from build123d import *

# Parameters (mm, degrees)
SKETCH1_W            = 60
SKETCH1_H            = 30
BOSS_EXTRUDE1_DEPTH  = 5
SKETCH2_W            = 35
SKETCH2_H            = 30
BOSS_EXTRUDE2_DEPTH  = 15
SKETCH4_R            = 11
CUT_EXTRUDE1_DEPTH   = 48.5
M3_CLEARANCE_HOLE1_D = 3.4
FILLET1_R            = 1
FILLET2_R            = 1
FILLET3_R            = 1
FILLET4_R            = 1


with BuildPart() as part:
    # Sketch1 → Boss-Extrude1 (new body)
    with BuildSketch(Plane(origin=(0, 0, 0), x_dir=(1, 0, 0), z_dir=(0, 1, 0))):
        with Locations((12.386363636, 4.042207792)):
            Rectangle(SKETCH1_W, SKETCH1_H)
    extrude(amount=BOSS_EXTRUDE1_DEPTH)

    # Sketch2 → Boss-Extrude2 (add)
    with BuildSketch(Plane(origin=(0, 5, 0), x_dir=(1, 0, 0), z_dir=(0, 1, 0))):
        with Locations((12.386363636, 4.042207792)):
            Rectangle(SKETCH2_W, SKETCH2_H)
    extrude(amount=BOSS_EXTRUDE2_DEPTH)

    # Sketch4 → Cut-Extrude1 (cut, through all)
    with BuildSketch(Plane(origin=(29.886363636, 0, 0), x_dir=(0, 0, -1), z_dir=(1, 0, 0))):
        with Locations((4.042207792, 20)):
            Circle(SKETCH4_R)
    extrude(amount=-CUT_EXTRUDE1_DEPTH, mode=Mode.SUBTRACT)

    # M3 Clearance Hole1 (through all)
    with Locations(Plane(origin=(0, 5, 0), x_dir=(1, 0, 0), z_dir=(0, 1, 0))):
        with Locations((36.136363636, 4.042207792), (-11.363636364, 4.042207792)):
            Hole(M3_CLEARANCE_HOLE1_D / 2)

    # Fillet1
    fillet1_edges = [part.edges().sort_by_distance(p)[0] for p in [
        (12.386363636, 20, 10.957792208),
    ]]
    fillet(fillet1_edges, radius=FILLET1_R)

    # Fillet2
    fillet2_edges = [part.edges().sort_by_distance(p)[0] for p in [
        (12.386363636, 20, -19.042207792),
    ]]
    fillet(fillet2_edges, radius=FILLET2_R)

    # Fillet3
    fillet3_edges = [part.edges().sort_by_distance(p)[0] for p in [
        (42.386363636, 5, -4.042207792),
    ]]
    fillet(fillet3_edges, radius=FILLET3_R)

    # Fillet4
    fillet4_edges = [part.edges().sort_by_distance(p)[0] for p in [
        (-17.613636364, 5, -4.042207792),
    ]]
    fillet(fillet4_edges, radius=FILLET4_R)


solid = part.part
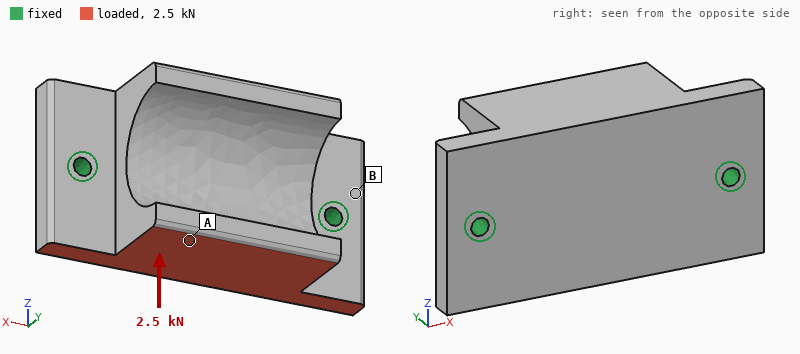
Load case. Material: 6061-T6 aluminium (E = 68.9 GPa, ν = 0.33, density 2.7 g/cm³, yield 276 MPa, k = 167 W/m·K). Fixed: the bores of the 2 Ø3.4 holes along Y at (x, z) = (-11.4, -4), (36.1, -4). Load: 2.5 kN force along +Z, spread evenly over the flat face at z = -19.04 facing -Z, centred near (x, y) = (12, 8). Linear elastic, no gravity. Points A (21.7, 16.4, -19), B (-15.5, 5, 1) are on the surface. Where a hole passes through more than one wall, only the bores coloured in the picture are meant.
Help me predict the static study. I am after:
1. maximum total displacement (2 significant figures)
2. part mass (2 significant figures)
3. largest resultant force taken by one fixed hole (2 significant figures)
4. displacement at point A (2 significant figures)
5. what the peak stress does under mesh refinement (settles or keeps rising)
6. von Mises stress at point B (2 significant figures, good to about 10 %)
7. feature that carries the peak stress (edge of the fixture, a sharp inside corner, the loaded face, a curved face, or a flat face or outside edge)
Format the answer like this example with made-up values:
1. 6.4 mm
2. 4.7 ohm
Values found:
1. 74 µm
2. 49 g
3. 1.3 kN
4. 65 µm
5. keeps rising
6. 30 MPa
7. edge of the fixture
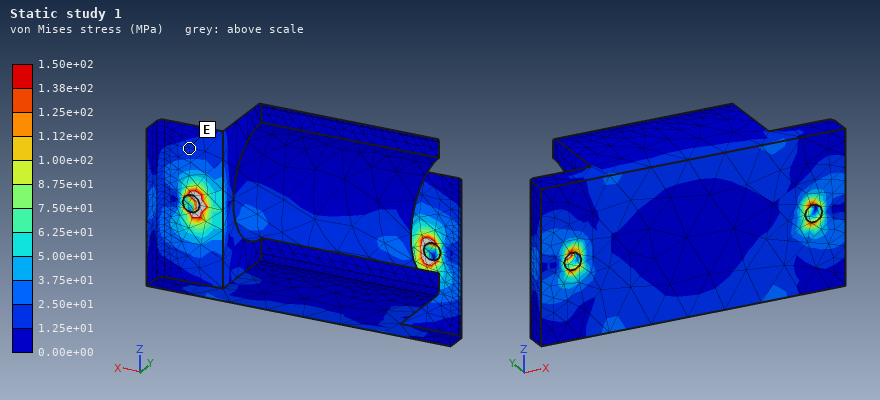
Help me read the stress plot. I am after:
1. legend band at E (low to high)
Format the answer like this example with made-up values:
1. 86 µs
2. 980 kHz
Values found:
1. 1.25e+01 to 2.50e+01 MPa
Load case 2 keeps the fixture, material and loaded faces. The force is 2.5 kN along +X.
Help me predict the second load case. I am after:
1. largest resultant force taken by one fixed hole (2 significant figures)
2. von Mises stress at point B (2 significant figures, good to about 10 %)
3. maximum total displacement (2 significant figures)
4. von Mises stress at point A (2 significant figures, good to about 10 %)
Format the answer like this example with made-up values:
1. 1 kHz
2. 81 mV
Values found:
1. 1.5 kN
2. 6.1 MPa
3. 11 µm
4. 8.3 MPa
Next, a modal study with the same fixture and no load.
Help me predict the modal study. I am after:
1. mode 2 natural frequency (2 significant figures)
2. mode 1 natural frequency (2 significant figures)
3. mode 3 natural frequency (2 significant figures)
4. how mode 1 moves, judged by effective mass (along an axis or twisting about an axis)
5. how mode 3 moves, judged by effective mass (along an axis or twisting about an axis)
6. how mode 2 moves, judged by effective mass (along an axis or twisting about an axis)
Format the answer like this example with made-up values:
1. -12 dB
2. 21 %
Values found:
1. 9600 Hz
2. 4900 Hz
3. 16 kHz
4. along Z
5. along X
6. along Y
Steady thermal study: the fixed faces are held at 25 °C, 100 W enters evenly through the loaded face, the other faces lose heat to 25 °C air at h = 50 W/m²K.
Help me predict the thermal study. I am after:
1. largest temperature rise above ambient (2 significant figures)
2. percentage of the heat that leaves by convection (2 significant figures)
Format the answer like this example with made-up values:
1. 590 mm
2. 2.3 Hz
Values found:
1. 45 K
2. 6.4 %
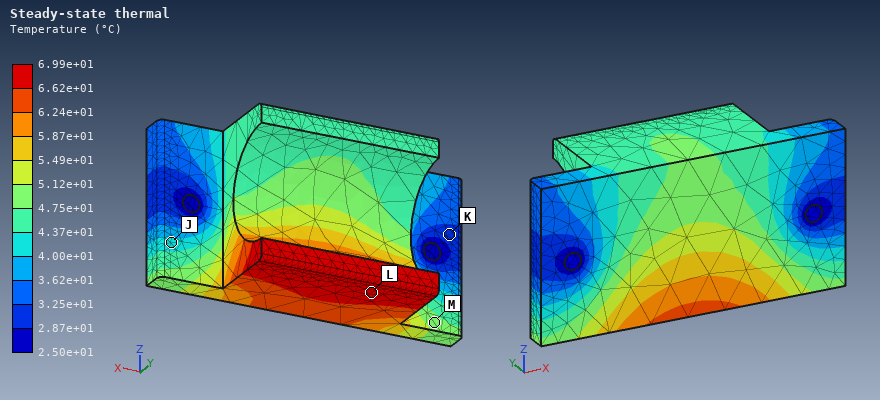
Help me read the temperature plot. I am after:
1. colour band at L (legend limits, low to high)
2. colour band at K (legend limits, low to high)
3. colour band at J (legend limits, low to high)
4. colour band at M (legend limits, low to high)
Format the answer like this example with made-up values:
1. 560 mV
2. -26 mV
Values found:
1. 6.62e+01 to 6.99e+01 °C
2. 2.87e+01 to 3.25e+01 °C
3. 4.00e+01 to 4.37e+01 °C
4. 4.75e+01 to 5.12e+01 °C
